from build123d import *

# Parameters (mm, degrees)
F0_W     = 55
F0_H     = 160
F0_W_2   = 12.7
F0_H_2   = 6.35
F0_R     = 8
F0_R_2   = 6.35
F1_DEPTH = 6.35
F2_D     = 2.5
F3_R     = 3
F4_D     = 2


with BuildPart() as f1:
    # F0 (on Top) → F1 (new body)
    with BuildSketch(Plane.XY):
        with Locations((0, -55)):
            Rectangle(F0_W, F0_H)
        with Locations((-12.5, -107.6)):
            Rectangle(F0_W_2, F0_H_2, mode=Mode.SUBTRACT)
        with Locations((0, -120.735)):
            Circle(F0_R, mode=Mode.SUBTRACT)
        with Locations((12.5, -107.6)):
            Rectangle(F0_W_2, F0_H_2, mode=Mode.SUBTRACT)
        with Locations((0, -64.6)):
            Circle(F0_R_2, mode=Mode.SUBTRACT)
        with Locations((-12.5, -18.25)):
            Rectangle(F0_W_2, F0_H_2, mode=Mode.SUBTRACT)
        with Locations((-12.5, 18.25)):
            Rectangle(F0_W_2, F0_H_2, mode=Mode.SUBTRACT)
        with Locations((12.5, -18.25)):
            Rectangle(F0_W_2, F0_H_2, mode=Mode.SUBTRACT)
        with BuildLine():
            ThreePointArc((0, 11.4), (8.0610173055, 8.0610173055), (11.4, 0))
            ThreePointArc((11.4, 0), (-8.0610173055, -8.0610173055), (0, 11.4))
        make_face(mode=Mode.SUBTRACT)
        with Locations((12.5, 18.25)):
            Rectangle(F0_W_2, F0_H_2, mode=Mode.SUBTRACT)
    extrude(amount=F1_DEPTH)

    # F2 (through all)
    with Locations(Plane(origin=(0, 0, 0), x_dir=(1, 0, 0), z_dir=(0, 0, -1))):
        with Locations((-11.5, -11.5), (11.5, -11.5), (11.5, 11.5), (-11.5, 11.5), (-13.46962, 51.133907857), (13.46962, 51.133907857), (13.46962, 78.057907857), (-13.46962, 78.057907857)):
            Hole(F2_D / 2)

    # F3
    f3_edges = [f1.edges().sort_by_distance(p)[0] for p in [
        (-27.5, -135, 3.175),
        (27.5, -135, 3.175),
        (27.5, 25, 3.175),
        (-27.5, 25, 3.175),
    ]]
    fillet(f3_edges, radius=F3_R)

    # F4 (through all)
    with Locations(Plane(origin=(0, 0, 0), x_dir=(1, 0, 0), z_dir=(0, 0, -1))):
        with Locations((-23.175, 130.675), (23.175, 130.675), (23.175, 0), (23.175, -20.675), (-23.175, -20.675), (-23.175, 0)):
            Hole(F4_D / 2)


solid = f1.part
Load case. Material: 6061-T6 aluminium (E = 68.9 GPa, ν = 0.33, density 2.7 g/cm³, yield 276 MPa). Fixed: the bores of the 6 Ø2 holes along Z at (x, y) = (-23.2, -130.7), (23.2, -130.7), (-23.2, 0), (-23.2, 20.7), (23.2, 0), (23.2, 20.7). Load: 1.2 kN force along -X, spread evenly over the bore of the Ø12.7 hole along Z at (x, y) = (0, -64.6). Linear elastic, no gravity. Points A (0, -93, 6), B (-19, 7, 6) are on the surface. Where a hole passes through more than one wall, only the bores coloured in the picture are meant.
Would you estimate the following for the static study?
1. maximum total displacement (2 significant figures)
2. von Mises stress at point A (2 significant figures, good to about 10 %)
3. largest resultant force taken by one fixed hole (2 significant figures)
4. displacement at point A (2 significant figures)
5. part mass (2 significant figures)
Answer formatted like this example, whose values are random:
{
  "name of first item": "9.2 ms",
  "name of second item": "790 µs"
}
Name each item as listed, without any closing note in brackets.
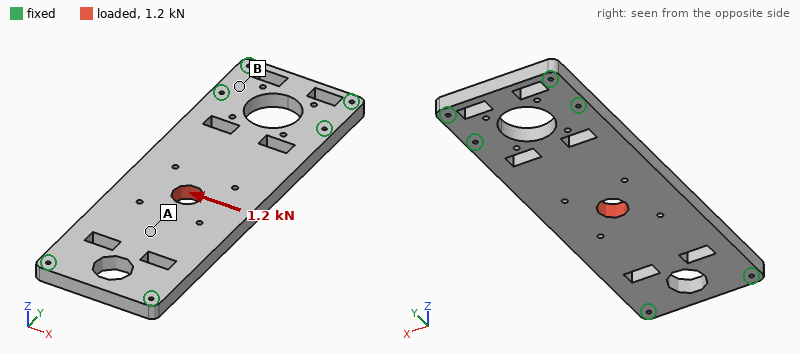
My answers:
{
  "maximum total displacement": "11 µm",
  "von Mises stress at point A": "3.2 MPa",
  "largest resultant force taken by one fixed hole": "490 N",
  "displacement at point A": "8.0 µm",
  "part mass": "130 g"
}
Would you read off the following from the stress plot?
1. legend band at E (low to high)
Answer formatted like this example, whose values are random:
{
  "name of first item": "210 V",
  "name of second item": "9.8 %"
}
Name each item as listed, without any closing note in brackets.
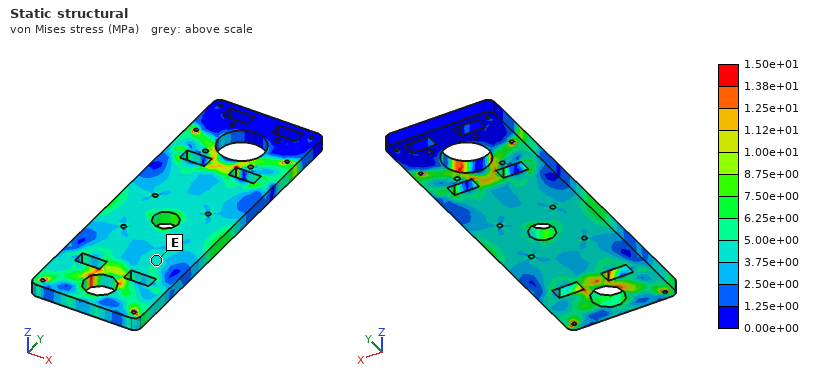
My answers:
{
  "legend band at E": "3.75e+00 to 5.00e+00 MPa"
}
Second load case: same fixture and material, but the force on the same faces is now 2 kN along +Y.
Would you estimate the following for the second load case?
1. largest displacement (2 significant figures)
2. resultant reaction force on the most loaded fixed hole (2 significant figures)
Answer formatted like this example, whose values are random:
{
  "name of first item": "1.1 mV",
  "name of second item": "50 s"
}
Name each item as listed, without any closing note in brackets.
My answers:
{
  "largest displacement": "5.7 µm",
  "resultant reaction force on the most loaded fixed hole": "500 N"
}
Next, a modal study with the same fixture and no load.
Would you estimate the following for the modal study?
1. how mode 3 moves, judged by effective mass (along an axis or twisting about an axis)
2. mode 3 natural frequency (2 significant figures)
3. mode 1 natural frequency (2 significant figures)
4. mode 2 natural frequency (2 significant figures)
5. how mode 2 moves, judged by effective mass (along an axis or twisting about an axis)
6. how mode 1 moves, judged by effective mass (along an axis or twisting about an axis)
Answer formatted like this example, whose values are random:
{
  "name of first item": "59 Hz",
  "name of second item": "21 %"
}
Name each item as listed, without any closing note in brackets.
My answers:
{
  "how mode 3 moves, judged by effective mass": "twisting about X",
  "mode 3 natural frequency": "4300 Hz",
  "mode 1 natural frequency": "1500 Hz",
  "mode 2 natural frequency": "3000 Hz",
  "how mode 2 moves, judged by effective mass": "twisting about Y",
  "how mode 1 moves, judged by effective mass": "along Z"
}
